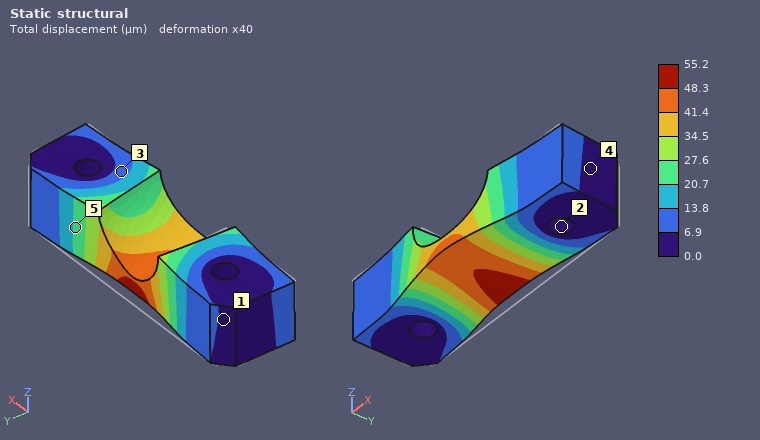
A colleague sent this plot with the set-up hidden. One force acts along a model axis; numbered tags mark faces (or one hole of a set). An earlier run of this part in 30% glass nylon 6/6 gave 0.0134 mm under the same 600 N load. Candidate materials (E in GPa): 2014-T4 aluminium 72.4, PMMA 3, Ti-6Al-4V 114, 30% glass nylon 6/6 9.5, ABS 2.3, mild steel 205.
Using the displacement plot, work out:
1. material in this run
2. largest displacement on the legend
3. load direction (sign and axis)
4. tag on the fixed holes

ABS
55.2 µm
-Y
2
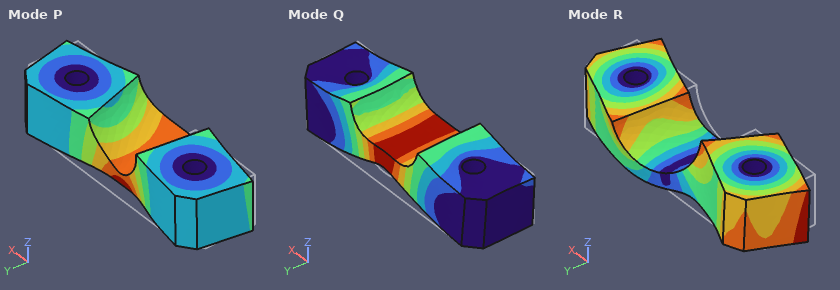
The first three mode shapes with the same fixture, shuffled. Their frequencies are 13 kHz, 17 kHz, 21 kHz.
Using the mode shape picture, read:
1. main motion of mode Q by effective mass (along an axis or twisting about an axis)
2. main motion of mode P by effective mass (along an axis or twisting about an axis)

along Z
along Y
